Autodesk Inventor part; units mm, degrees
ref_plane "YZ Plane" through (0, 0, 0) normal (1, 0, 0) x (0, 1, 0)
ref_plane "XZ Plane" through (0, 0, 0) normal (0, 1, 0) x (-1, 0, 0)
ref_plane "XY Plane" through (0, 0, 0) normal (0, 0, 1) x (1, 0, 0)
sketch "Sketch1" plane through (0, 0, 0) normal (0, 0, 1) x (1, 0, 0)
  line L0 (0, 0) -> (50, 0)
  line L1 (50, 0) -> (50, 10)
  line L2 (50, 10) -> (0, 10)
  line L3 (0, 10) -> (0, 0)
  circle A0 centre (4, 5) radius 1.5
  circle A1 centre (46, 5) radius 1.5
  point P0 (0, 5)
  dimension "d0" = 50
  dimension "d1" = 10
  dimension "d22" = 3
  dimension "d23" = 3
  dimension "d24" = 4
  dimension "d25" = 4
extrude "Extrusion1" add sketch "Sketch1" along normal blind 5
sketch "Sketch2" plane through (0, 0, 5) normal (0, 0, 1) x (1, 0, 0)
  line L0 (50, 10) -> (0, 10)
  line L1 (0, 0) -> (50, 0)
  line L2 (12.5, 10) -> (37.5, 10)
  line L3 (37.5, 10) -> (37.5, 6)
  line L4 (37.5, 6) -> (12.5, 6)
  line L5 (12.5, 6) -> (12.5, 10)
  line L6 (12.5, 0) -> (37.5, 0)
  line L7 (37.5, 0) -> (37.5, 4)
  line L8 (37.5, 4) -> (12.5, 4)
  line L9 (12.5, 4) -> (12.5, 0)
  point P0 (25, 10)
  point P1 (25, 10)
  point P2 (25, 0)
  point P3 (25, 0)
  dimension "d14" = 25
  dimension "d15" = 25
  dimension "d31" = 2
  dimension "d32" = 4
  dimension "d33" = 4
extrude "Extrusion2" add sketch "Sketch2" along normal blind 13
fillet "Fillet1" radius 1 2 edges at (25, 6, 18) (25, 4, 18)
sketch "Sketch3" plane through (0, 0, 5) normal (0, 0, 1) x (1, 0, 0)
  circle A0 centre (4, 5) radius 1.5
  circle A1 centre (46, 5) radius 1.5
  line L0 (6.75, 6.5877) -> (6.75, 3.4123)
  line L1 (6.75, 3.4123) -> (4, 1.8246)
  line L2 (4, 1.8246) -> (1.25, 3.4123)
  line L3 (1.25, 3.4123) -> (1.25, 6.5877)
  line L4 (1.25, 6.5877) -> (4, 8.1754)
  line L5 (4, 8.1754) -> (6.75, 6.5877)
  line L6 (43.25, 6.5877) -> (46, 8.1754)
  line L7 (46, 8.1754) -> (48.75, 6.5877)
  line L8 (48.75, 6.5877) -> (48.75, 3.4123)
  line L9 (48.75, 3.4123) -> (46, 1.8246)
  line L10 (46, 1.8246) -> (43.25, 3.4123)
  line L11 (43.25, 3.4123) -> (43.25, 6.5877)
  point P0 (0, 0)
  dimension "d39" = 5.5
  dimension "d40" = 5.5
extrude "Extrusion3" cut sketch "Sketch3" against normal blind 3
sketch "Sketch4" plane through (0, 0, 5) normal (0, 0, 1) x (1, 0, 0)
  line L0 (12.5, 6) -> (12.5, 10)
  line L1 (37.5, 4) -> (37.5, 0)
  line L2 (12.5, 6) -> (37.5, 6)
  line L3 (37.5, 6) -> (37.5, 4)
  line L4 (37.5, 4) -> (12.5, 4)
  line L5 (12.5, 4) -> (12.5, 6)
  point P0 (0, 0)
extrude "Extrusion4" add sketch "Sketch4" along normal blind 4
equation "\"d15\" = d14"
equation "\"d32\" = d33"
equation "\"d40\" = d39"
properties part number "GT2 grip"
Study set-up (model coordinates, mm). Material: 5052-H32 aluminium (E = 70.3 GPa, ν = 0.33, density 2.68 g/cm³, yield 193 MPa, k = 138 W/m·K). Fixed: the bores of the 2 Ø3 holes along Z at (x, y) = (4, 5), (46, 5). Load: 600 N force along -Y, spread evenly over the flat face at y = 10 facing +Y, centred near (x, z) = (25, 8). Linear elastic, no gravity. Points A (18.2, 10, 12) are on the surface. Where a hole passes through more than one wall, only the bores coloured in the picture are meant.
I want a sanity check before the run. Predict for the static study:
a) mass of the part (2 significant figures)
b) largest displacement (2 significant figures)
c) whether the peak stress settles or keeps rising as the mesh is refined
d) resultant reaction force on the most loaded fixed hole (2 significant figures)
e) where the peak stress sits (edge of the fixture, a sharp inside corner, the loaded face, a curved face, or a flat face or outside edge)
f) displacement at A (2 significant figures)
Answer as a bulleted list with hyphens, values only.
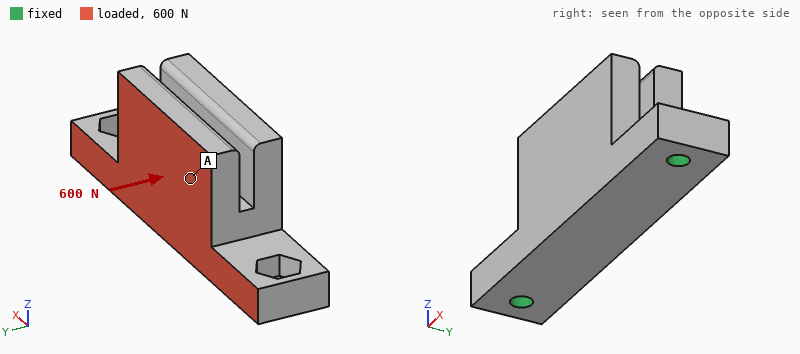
- 14 g
- 93 µm
- keeps rising
- 300 N
- edge of the fixture
- 63 µm
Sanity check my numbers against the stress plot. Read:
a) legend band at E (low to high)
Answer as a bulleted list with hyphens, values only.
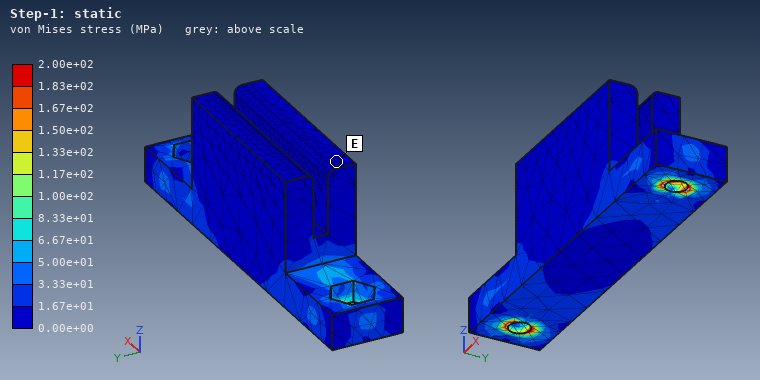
- 0.00e+00 to 1.67e+01 MPa
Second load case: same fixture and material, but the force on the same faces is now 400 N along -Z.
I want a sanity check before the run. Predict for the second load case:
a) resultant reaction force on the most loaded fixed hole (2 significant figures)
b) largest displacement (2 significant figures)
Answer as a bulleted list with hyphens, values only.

- 270 N
- 43 µm
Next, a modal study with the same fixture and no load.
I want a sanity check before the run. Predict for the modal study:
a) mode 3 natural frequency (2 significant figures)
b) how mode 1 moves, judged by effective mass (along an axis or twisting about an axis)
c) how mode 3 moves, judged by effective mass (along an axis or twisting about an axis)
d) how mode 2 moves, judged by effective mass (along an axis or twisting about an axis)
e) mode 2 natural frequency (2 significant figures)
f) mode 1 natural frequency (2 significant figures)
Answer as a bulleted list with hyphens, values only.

- 17 kHz
- along Y
- along Y
- along Z
- 11 kHz
- 4400 Hz
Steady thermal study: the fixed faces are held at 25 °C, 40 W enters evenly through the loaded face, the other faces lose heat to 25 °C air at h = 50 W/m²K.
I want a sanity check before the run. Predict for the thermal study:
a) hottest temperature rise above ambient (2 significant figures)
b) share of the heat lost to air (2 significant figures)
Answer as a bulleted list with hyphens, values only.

- 44 K
- 8.4 %
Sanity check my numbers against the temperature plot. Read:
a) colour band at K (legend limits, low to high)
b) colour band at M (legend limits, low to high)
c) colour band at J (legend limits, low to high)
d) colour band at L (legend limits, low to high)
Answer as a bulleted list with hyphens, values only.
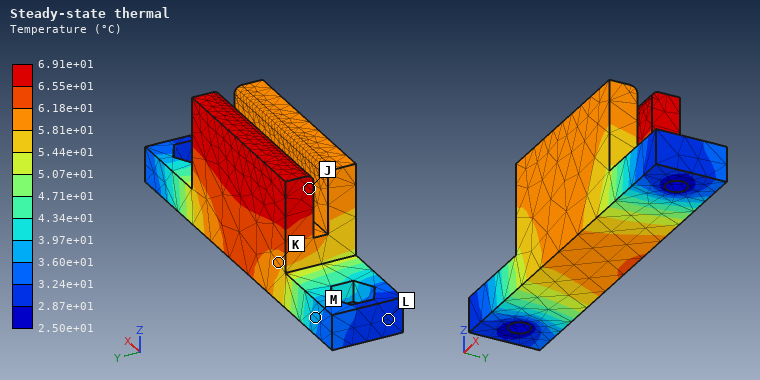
- 5.81e+01 to 6.18e+01 °C
- 3.60e+01 to 3.97e+01 °C
- 6.55e+01 to 6.91e+01 °C
- 2.87e+01 to 3.24e+01 °C
